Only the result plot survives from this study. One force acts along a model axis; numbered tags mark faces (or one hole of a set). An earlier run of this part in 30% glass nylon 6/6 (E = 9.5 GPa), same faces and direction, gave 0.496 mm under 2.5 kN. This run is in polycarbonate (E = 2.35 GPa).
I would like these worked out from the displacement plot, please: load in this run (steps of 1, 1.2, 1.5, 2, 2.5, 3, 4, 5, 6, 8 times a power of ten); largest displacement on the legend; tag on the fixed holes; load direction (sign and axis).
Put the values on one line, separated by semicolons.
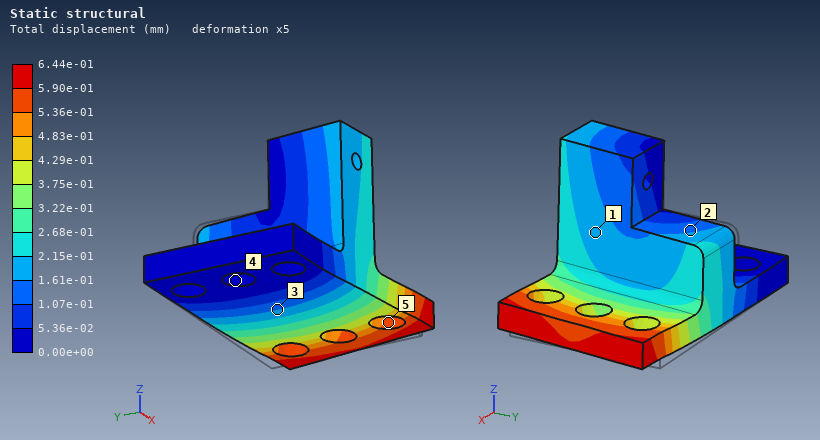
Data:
800 N; 6.44e-01 mm; 4; -Y
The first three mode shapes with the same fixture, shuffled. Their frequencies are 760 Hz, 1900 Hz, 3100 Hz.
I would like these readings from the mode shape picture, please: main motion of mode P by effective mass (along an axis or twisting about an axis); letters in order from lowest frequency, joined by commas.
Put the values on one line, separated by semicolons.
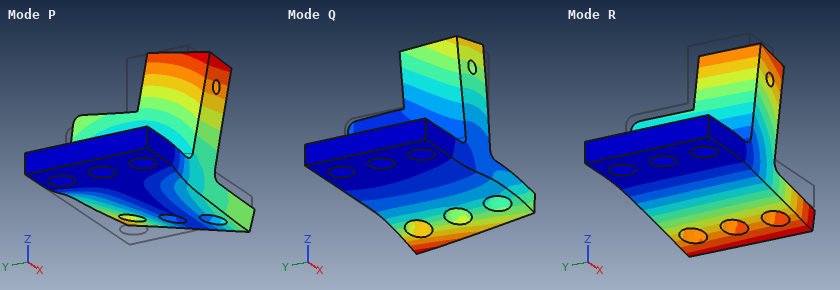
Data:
along Y; R, P, Q
